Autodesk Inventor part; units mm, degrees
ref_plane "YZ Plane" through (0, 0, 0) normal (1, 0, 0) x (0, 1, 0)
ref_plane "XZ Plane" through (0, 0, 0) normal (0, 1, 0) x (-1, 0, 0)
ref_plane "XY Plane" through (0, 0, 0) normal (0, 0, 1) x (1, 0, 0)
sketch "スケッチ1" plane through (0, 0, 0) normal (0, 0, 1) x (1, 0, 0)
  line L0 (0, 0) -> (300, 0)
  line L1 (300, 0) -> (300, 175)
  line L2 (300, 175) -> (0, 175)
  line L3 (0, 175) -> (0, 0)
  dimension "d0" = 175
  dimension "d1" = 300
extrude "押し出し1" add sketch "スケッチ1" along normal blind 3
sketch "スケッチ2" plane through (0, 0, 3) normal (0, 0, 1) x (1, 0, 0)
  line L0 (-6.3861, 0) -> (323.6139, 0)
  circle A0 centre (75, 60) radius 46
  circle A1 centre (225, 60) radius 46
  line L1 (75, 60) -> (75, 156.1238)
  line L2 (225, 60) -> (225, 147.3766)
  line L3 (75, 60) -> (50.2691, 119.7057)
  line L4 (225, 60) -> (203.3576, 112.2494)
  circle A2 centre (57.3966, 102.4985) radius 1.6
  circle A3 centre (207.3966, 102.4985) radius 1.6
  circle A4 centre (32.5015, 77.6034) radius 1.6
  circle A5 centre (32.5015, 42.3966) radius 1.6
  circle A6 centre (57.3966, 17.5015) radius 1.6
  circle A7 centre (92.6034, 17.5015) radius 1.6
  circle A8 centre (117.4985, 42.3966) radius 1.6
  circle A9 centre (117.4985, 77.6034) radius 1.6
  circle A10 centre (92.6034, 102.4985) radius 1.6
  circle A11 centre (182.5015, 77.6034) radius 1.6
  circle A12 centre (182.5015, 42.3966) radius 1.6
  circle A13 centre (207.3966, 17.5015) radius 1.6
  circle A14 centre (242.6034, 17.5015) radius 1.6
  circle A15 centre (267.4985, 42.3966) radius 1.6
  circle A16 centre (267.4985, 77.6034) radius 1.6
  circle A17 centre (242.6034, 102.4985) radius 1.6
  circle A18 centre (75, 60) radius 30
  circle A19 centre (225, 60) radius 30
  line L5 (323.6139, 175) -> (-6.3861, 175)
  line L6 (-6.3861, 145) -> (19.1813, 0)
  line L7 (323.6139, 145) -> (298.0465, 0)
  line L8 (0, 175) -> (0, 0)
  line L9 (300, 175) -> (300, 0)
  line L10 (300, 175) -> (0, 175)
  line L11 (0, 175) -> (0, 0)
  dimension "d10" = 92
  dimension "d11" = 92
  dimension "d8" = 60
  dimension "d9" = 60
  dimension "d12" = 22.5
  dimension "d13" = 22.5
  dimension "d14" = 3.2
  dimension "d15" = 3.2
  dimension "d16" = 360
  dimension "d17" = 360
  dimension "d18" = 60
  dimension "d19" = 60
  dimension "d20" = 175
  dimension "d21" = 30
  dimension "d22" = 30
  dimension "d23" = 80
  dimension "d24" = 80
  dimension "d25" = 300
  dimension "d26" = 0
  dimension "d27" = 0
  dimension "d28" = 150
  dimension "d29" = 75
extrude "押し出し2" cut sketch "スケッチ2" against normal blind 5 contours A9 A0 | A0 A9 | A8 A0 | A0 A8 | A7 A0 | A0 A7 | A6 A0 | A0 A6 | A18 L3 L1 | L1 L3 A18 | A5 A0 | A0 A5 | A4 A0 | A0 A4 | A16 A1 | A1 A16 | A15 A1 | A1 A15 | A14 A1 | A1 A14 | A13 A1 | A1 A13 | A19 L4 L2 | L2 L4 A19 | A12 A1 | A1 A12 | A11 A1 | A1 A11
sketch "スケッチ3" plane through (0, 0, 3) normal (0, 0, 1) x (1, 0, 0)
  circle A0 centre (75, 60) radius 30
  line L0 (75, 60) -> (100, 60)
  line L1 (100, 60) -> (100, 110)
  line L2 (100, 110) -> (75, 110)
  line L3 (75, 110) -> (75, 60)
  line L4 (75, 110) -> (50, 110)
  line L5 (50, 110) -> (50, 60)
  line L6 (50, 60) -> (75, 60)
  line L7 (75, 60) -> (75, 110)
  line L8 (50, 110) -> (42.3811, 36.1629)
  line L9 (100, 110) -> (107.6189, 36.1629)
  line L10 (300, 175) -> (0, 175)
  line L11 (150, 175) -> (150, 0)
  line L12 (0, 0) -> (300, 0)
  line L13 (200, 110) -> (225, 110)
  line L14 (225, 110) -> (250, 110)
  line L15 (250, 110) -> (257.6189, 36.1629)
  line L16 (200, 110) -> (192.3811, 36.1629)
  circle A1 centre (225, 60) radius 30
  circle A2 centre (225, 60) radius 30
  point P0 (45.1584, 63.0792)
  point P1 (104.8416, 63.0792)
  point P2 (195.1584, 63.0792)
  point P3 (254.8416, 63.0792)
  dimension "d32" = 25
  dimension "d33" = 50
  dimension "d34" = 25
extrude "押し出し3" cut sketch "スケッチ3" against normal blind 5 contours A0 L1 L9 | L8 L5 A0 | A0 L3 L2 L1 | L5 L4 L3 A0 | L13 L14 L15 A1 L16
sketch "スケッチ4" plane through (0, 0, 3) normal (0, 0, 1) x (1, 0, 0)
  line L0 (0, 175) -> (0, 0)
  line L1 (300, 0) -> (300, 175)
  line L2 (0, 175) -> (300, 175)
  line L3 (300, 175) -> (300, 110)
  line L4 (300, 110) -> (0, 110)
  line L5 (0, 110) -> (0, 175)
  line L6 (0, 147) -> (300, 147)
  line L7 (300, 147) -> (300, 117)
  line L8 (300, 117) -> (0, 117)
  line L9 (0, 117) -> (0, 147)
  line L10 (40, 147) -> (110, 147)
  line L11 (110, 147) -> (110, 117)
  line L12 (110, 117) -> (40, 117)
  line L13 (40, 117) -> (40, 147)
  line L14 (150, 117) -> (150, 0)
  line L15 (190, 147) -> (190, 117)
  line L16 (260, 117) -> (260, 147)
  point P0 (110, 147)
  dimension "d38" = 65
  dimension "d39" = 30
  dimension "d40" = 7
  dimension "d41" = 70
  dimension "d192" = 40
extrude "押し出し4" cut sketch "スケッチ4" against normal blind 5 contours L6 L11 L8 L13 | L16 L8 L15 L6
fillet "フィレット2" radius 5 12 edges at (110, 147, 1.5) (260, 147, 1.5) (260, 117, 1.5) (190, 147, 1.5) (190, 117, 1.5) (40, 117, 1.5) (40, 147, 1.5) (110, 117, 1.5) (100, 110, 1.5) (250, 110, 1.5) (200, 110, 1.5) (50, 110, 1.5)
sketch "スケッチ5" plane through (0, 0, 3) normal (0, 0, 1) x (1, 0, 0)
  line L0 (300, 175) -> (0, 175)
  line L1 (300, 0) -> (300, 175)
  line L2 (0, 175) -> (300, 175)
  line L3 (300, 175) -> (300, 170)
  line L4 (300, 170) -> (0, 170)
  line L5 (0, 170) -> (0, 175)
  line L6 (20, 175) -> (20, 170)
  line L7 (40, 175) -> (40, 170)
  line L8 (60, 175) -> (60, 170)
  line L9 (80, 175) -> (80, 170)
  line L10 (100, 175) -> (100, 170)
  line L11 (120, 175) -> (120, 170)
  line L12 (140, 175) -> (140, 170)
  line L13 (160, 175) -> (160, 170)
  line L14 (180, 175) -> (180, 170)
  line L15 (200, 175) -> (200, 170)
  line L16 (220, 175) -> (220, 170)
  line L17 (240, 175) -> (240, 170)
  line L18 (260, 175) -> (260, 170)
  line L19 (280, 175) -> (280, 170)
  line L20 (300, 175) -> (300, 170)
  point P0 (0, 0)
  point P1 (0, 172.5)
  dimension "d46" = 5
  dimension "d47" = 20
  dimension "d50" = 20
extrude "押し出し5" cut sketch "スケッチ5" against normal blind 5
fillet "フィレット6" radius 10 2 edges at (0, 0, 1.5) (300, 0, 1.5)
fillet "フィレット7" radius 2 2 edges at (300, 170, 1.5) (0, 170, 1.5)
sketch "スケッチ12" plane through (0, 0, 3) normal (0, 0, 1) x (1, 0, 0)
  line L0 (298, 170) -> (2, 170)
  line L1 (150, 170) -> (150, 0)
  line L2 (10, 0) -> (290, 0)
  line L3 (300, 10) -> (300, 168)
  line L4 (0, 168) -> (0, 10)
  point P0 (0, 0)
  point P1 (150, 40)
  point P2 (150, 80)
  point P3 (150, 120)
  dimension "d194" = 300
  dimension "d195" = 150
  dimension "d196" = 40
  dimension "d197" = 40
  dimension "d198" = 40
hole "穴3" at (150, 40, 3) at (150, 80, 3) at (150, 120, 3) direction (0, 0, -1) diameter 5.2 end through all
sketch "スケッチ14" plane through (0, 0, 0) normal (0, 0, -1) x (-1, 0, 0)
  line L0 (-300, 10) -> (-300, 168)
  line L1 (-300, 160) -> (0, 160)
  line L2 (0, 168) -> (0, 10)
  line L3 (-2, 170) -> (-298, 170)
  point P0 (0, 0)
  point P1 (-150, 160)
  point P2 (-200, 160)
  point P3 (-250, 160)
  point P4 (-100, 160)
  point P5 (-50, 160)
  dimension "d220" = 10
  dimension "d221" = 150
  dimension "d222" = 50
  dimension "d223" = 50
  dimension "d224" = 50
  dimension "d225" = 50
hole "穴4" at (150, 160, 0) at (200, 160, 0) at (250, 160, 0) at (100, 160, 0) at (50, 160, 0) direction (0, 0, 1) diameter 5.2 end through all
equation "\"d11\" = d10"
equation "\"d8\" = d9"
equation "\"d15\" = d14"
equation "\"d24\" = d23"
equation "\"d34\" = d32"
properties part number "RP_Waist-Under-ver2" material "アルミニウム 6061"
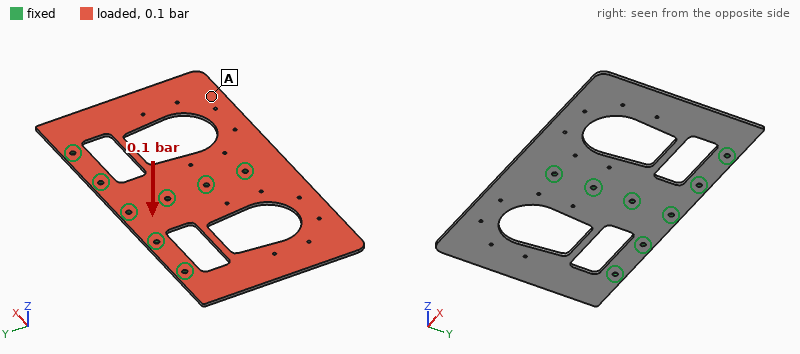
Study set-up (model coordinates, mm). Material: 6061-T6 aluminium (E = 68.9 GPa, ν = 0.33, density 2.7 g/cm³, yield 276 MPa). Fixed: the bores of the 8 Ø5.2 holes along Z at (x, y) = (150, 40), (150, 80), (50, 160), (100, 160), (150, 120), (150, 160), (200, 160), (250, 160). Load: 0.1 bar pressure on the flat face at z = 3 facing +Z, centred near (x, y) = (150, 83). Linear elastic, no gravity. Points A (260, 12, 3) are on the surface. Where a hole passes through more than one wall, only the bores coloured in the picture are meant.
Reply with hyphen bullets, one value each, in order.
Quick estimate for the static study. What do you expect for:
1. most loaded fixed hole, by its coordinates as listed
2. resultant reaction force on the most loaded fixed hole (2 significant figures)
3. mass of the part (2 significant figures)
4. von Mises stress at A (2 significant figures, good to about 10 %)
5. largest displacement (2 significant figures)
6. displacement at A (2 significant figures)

- (150, 40)
- 180 N
- 310 g
- 8.4 MPa
- 2.3 mm
- 1.5 mm
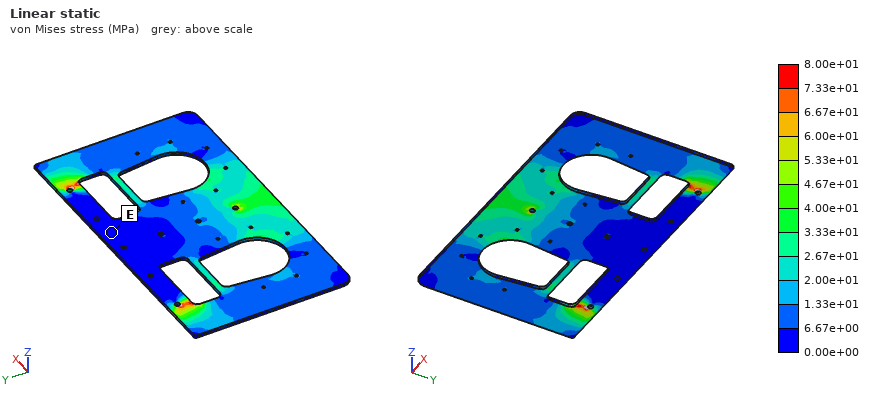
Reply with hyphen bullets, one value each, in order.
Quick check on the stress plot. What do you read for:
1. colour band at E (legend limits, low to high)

- 0.00e+00 to 6.67e+00 MPa
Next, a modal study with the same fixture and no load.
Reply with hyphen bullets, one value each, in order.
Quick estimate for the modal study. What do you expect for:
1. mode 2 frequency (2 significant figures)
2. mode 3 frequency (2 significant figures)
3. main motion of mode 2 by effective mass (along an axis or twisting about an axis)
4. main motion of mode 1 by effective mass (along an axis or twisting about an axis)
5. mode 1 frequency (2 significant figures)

- 160 Hz
- 480 Hz
- along Z
- twisting about Y
- 150 Hz
